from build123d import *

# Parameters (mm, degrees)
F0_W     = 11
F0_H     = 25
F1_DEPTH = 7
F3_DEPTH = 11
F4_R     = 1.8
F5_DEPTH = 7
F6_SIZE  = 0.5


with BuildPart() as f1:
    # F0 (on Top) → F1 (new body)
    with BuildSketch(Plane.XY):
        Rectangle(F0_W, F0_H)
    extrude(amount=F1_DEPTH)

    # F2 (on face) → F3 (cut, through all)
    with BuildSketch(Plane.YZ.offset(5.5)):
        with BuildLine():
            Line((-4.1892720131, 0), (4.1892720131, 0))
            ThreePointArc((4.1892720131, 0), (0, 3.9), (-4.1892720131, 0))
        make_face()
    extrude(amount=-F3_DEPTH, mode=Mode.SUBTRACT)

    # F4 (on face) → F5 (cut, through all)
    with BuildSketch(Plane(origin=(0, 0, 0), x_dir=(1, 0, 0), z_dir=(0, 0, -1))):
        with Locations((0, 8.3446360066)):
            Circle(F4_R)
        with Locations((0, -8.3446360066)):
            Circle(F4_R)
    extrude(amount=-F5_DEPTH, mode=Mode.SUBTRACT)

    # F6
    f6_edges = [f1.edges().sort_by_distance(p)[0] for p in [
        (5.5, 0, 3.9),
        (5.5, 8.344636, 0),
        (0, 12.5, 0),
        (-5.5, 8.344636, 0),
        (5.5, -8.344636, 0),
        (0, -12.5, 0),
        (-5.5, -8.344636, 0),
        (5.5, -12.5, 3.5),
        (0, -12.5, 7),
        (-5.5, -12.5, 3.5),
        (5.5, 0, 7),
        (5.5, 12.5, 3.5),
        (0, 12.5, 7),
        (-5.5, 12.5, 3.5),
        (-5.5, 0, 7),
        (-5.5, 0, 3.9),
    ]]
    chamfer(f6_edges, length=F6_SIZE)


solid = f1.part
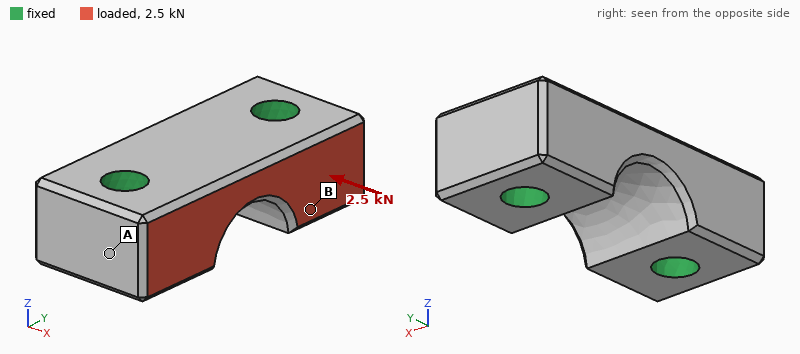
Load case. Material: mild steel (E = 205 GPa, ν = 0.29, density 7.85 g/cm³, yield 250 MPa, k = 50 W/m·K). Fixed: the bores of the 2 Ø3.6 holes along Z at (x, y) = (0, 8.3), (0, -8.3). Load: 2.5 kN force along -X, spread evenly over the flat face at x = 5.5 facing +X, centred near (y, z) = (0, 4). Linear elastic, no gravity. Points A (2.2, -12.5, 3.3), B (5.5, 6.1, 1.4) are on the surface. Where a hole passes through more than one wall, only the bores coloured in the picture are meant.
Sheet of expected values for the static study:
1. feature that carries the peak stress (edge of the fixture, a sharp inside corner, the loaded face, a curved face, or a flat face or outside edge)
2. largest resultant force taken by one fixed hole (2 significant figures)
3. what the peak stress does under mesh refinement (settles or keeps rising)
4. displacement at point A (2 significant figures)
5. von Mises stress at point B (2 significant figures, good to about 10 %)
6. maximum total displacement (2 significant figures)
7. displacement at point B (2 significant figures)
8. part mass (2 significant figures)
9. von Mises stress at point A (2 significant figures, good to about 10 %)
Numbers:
edge of the fixture
1.3 kN
keeps rising
0.19 µm
20 MPa
1.1 µm
0.60 µm
12 g
9.5 MPa
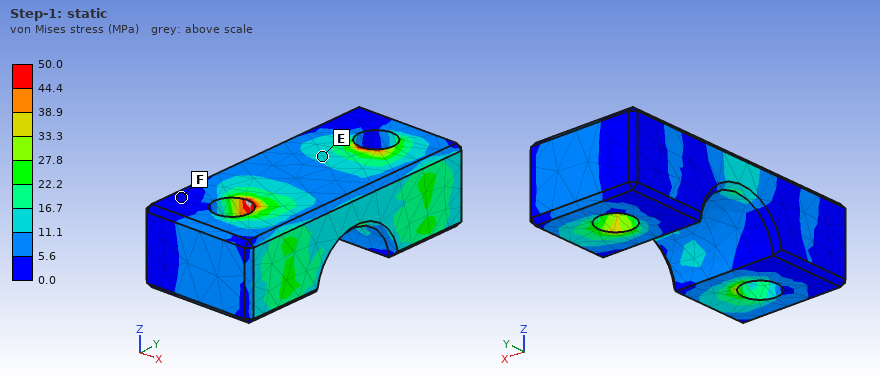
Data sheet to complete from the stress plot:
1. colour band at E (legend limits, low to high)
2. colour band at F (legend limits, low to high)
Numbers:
11.1 to 16.7 MPa
0.0 to 5.6 MPa
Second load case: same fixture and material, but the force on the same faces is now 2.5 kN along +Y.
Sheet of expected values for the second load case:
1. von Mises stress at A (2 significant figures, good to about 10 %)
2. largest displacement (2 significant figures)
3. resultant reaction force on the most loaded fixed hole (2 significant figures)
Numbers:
35 MPa
2.2 µm
1.3 kN
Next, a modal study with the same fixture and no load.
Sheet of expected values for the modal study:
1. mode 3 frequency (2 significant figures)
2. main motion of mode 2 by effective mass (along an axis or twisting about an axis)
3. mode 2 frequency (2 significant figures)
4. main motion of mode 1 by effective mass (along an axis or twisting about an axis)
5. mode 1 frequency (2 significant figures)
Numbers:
100 kHz
along Z
89 kHz
along X
81 kHz
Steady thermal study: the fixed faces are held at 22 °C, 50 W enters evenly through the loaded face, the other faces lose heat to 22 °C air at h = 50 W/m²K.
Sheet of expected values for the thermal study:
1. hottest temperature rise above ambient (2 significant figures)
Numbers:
42 K
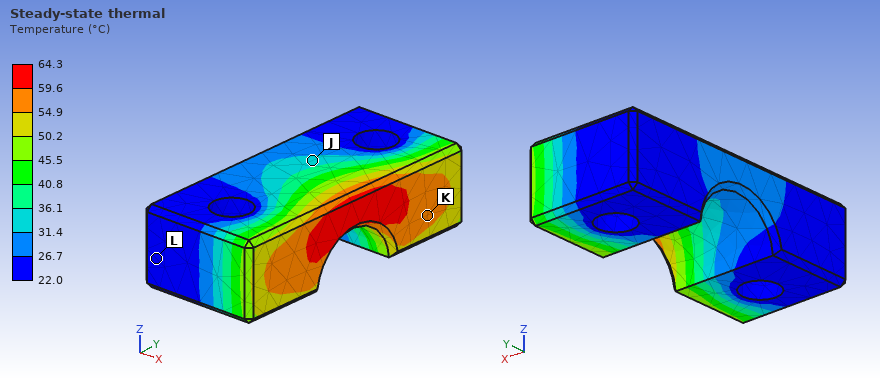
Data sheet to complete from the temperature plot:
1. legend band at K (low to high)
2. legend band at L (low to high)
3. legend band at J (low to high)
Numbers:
54.9 to 59.6 °C
22.0 to 26.7 °C
31.4 to 36.1 °C
